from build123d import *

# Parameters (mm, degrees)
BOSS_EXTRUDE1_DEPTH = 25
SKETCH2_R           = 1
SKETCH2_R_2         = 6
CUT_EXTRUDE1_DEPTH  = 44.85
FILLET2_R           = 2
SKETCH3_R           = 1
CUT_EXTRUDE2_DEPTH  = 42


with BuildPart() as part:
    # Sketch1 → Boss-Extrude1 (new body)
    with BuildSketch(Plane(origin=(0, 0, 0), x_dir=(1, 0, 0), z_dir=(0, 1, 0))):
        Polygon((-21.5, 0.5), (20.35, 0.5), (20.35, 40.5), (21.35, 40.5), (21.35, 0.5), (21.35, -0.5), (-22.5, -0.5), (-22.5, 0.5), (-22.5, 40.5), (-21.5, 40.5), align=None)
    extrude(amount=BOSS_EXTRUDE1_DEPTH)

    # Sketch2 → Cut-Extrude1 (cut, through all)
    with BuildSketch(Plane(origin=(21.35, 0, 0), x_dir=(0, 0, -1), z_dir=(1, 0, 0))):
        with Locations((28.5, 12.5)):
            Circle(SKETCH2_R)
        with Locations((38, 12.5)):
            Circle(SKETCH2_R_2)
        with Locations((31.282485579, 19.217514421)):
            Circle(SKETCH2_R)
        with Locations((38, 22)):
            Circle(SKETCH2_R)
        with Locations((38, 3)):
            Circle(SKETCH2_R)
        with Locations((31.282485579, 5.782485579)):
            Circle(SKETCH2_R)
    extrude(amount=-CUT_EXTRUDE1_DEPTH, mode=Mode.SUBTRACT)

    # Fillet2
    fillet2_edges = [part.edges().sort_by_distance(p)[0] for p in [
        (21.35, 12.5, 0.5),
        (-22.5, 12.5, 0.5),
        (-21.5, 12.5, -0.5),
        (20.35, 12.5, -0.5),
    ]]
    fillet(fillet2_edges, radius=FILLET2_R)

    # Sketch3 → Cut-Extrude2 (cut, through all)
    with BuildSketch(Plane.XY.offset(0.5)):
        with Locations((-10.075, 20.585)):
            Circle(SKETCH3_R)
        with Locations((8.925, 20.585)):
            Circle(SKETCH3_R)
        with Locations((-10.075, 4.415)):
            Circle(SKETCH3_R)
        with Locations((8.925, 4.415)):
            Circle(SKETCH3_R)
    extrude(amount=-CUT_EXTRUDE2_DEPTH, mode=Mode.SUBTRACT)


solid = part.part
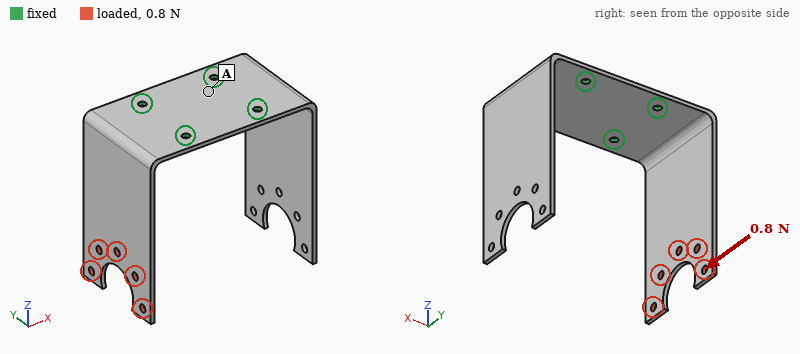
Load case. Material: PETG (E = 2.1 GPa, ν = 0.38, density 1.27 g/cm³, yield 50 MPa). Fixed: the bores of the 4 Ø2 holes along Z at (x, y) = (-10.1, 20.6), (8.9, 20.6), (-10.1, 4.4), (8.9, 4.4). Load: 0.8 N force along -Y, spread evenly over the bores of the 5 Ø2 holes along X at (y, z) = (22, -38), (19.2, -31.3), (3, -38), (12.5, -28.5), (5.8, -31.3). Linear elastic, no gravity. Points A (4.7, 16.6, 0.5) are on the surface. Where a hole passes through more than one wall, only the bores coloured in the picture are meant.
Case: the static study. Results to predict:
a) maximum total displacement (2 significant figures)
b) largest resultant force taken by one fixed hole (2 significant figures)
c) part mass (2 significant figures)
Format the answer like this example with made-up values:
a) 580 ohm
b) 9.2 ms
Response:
a) 0.68 mm
b) 1.7 N
c) 3.7 g
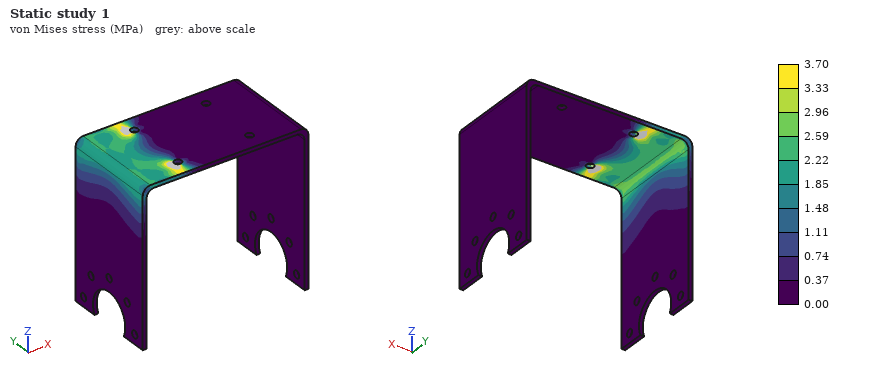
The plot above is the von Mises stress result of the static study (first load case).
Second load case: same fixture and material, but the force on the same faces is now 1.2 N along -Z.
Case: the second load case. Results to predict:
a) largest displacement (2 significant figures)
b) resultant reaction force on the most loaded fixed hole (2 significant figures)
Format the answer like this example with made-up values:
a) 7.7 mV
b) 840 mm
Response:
a) 0.73 mm
b) 0.66 N
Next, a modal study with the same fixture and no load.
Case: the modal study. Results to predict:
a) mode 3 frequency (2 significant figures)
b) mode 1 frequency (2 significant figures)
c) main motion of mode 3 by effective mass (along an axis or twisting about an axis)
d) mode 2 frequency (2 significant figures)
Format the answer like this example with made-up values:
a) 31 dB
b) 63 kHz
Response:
a) 260 Hz
b) 110 Hz
c) along Y
d) 110 Hz
